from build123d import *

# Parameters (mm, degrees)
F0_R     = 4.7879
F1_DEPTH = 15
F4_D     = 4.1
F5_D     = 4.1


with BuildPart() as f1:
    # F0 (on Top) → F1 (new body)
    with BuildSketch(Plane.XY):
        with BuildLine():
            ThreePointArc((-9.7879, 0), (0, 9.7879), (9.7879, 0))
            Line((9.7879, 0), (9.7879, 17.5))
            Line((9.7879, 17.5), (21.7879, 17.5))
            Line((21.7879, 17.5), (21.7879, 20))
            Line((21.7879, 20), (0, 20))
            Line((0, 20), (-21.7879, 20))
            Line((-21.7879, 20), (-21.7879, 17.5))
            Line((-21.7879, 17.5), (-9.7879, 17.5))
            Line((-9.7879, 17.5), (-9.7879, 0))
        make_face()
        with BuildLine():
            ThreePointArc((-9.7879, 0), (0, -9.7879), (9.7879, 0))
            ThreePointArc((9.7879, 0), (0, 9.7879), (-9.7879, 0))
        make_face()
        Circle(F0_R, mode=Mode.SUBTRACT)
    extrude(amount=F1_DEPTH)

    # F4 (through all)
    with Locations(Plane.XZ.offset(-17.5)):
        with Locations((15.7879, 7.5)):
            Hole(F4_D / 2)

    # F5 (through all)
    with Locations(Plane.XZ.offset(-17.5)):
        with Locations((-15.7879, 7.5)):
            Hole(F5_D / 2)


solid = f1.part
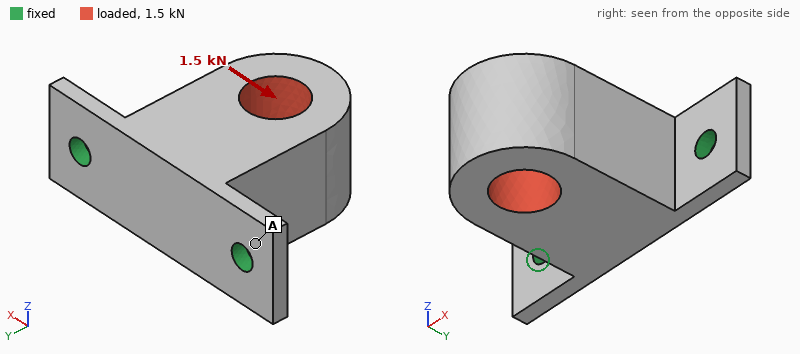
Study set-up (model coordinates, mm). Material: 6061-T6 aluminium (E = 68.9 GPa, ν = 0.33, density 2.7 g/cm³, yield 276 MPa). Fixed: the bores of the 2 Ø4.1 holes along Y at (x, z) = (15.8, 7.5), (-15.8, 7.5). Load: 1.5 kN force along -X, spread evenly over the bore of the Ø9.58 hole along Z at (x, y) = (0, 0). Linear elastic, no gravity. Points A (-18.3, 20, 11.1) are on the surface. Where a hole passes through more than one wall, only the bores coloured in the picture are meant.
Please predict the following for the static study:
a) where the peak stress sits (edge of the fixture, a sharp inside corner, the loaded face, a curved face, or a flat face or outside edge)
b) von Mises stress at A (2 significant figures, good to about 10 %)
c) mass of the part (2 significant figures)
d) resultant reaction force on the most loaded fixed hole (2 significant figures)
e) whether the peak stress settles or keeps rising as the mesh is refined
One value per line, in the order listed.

edge of the fixture
38 MPa
21 g
1.4 kN
keeps rising
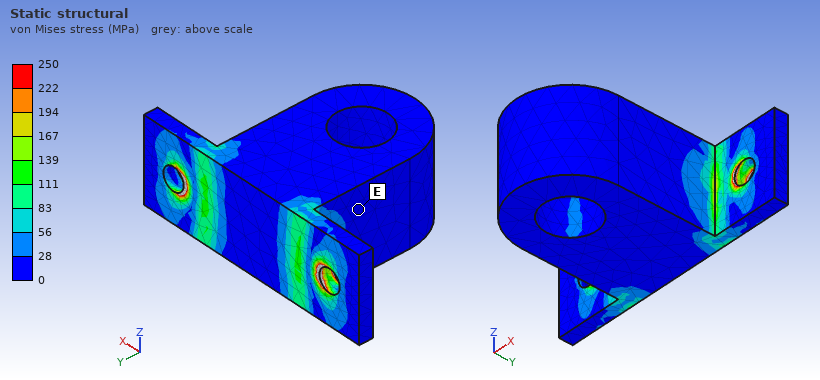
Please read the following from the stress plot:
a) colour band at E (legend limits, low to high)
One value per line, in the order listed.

0 to 28 MPa
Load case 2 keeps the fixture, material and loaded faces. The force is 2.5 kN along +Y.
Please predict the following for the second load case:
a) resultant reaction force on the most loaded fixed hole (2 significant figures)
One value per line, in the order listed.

1.4 kN
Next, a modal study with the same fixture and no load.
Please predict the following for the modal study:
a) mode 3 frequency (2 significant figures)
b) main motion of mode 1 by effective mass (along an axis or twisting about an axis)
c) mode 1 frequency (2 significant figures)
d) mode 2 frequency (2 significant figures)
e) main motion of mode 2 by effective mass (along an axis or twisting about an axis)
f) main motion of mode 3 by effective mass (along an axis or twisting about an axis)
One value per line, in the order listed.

9600 Hz
along Z
2400 Hz
7200 Hz
along X
along Y
